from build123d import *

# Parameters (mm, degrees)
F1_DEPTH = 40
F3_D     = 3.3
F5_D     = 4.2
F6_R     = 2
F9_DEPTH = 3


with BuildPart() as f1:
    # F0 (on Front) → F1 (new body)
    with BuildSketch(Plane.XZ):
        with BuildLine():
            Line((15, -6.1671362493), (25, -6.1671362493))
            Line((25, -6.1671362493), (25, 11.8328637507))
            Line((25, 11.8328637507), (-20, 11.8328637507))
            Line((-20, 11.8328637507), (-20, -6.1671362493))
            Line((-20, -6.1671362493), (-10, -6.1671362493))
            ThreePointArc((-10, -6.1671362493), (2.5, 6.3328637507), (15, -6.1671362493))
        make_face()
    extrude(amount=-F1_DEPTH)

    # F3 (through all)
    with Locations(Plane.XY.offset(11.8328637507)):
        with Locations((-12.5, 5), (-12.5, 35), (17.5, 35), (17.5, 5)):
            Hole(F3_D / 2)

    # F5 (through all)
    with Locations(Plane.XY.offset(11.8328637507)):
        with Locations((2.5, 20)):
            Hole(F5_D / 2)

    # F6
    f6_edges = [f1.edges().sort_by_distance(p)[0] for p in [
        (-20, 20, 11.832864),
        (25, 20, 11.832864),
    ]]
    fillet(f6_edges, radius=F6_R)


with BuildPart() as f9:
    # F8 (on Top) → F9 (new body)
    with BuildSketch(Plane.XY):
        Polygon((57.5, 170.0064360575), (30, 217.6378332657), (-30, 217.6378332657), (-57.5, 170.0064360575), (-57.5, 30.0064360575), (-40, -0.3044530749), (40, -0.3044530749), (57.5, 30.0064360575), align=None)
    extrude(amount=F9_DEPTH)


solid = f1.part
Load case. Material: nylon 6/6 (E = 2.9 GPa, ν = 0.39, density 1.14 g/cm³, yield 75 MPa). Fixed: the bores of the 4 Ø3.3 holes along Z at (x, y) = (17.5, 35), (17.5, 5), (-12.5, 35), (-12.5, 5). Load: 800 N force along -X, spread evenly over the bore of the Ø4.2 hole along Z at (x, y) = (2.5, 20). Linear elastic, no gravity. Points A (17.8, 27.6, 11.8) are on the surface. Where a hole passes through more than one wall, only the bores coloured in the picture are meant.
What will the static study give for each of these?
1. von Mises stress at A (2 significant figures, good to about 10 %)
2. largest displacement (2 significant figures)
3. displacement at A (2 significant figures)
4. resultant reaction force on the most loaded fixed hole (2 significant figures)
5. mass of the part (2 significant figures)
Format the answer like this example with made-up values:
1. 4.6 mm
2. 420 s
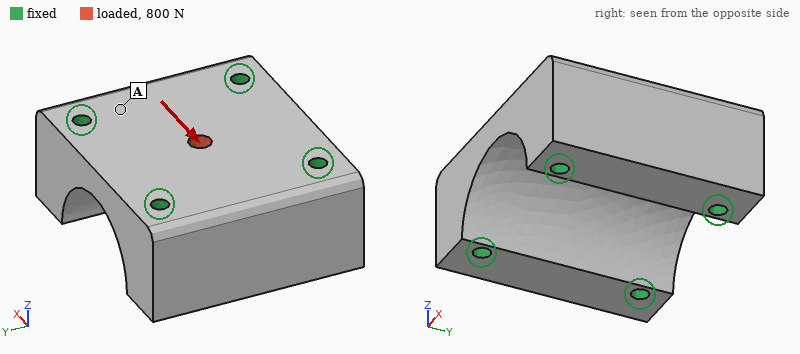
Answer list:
1. 1.8 MPa
2. 34 µm
3. 9.5 µm
4. 220 N
5. 25 g
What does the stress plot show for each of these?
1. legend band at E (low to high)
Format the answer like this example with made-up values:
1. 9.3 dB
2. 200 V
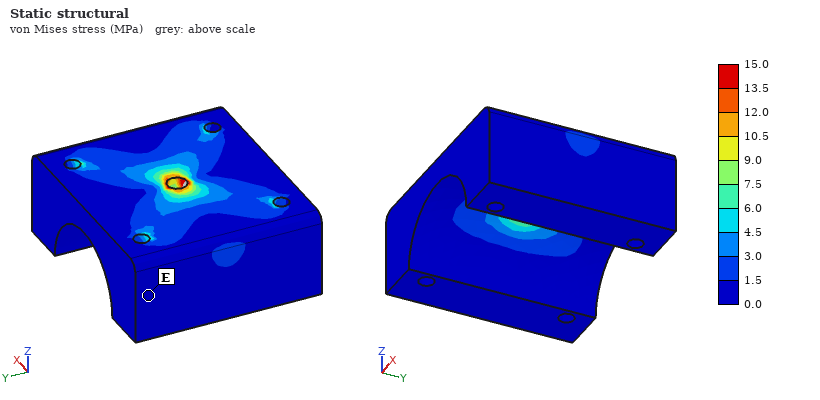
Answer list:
1. 0.0 to 1.5 MPa
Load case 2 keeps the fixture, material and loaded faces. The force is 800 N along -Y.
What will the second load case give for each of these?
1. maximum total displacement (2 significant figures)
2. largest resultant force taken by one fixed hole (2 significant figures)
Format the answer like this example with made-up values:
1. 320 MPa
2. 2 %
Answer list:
1. 35 µm
2. 240 N
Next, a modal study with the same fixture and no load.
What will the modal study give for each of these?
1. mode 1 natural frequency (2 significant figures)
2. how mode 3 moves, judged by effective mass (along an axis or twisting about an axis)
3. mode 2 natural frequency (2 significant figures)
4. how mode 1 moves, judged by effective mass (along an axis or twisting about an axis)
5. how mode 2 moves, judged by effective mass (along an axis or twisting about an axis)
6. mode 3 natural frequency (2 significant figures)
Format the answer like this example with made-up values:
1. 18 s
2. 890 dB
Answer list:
1. 11 kHz
2. along Z
3. 12 kHz
4. along Z
5. along X
6. 12 kHz
